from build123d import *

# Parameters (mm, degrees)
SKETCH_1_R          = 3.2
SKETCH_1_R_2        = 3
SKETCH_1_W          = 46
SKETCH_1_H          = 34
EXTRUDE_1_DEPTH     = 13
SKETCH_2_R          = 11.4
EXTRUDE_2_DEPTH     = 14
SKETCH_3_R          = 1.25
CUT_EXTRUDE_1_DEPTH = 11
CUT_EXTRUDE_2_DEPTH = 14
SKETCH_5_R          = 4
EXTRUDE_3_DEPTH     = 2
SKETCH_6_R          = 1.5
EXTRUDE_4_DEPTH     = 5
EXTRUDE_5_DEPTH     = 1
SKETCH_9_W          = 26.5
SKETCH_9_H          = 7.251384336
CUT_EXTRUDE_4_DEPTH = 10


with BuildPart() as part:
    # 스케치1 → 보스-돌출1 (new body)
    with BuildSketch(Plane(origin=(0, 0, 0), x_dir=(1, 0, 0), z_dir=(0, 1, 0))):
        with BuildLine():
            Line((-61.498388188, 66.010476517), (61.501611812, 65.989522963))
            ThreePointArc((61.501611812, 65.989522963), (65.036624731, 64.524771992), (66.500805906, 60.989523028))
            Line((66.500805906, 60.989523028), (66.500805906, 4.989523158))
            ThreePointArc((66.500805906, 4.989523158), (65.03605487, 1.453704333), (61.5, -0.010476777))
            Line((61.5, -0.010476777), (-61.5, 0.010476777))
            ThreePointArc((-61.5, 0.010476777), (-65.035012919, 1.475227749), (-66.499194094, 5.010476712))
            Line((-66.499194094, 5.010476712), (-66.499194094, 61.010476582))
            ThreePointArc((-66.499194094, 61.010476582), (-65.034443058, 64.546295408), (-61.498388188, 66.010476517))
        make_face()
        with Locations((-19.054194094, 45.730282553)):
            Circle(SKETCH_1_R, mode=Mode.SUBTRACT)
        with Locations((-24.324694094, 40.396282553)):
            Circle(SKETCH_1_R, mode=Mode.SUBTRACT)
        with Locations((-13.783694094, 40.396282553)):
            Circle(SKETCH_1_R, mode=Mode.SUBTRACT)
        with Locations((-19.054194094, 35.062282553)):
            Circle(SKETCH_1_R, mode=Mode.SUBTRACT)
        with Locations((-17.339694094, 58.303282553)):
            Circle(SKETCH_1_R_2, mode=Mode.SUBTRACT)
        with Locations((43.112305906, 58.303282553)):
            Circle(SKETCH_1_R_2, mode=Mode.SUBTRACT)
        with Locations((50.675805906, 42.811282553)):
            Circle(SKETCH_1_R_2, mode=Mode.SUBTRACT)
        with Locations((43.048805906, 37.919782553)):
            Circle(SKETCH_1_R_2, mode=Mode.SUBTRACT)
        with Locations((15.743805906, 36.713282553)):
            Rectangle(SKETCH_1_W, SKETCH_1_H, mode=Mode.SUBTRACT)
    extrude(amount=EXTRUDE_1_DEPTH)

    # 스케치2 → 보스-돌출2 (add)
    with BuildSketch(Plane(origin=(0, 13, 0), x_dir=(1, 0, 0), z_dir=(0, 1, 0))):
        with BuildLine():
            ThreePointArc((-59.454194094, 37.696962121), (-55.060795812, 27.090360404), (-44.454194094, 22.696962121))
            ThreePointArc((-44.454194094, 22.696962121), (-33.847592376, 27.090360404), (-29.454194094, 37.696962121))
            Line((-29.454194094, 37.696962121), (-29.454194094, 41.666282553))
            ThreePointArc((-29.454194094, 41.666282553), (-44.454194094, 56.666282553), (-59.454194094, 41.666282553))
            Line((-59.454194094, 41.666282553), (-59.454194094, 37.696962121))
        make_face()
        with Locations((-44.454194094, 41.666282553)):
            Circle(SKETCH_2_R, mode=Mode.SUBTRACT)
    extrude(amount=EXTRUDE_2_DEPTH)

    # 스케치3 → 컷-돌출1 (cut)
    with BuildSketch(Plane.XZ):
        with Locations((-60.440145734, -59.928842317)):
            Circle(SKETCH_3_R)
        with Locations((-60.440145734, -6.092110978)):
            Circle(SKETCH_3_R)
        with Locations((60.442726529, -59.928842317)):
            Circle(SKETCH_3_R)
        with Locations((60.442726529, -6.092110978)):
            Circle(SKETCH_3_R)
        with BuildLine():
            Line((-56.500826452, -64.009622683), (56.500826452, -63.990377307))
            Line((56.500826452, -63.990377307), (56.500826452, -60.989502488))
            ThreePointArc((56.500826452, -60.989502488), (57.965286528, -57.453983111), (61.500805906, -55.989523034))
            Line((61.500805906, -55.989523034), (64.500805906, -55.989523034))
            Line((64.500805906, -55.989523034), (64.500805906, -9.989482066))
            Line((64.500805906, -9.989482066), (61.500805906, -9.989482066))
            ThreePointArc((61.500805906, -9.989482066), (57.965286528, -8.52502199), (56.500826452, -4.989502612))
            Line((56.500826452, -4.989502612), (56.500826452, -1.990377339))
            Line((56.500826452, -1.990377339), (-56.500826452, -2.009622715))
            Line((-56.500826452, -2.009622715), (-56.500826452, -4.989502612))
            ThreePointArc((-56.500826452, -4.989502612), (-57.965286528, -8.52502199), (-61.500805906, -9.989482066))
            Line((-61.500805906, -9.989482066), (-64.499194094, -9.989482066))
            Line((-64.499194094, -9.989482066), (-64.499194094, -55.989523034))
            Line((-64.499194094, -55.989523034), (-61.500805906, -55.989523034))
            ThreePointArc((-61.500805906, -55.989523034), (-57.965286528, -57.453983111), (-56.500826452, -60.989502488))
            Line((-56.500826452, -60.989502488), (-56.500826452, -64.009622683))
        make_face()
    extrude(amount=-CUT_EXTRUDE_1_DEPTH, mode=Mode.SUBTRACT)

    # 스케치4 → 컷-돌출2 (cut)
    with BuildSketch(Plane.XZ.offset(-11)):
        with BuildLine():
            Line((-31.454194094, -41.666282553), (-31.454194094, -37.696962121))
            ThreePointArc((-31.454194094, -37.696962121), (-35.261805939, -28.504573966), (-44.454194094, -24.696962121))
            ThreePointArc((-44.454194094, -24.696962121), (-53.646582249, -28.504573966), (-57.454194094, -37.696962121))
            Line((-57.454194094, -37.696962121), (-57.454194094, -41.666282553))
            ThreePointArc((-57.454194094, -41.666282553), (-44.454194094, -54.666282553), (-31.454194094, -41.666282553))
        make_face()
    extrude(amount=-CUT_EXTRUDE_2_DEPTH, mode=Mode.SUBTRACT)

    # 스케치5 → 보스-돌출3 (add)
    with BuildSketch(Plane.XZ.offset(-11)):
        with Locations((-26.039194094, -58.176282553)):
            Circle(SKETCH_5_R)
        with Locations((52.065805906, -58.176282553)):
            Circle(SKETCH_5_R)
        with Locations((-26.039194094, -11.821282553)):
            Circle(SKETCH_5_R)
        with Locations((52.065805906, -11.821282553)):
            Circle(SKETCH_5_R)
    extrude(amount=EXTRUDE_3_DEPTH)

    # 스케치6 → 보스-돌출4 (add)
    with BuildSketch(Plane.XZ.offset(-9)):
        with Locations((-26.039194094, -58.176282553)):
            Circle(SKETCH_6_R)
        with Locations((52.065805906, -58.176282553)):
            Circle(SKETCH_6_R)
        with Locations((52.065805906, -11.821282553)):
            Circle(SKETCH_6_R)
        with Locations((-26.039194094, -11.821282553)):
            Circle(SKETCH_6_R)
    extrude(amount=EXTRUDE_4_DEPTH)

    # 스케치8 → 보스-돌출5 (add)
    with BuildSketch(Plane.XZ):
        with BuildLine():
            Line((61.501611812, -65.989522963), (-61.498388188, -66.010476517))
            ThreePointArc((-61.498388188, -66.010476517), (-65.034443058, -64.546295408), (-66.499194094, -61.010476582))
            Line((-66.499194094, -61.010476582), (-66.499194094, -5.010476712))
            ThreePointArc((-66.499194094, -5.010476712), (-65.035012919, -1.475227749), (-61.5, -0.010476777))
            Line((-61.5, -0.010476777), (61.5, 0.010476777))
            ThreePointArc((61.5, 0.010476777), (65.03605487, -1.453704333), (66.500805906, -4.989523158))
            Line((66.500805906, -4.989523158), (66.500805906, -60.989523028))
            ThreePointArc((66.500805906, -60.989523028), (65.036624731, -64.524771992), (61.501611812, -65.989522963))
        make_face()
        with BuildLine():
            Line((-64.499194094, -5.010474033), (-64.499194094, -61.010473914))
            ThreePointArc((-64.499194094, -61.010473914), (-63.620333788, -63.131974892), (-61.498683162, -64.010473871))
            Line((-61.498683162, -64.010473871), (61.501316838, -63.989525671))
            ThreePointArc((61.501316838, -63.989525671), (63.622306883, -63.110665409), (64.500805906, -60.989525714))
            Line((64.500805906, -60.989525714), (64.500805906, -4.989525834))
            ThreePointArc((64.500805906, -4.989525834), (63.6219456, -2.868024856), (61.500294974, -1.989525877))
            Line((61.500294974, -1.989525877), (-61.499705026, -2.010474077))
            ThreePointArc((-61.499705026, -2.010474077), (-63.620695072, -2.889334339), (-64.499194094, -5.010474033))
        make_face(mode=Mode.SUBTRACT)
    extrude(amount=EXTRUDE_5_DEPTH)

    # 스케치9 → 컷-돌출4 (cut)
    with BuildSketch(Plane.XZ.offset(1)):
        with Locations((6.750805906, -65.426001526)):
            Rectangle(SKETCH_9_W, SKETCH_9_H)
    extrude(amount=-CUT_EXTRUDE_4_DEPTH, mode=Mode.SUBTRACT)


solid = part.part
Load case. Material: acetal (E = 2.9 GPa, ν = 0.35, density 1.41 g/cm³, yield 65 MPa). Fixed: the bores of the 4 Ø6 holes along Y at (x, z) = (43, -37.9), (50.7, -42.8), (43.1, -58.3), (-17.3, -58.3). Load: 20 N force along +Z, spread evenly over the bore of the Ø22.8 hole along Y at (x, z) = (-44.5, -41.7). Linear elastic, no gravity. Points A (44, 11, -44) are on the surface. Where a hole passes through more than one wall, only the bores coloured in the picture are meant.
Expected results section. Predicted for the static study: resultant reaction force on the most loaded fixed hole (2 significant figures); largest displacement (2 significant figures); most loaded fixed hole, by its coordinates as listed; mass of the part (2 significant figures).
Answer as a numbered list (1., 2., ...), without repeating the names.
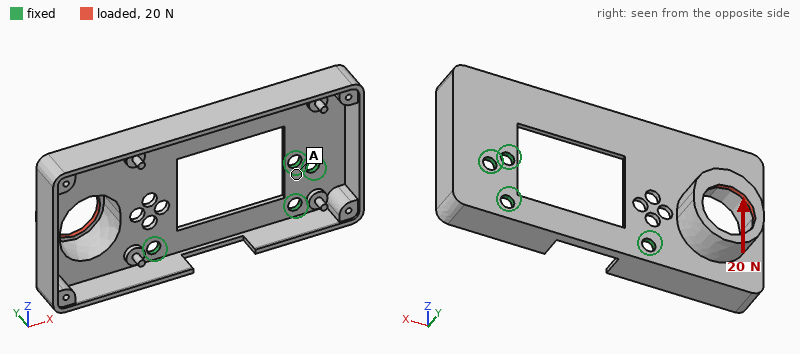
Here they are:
1. 22 N
2. 1.6 mm
3. (-17.3, -58.3)
4. 38 g
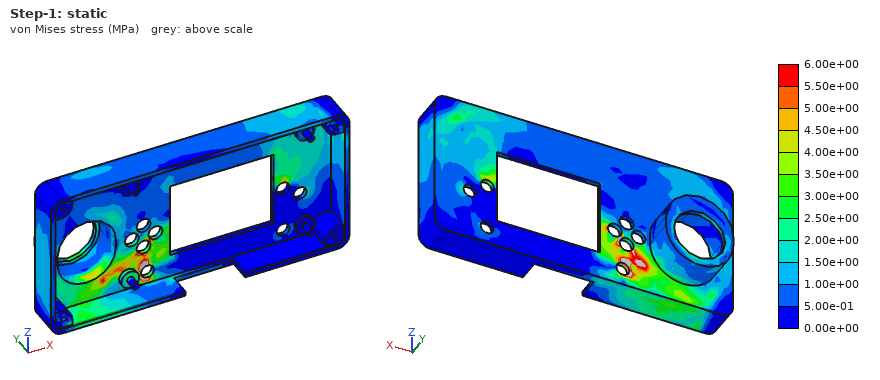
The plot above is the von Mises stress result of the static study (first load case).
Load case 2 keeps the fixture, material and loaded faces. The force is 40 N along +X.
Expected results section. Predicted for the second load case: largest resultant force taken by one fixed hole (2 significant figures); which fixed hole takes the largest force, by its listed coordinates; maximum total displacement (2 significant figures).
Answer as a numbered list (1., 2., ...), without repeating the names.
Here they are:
1. 35 N
2. (-17.3, -58.3)
3. 1.6 mm
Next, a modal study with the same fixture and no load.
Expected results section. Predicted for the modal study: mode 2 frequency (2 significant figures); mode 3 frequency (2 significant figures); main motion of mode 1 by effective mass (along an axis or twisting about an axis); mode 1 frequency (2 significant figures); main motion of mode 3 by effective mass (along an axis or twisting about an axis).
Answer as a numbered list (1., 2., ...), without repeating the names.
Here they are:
1. 300 Hz
2. 400 Hz
3. along Y
4. 100 Hz
5. along Y
